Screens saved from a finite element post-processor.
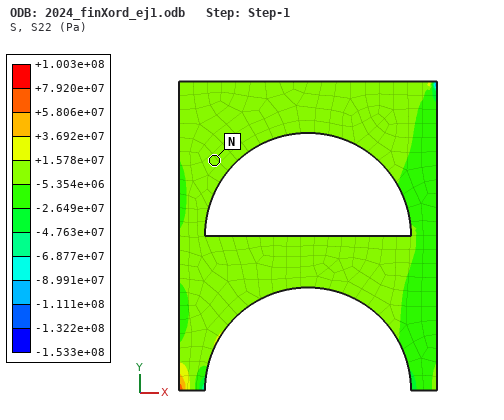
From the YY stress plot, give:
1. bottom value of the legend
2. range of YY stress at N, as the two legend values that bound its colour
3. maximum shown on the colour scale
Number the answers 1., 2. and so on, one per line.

1. -1.533e+08 Pa
2. -5.354e+06 to +1.578e+07 Pa
3. +1.003e+08 Pa
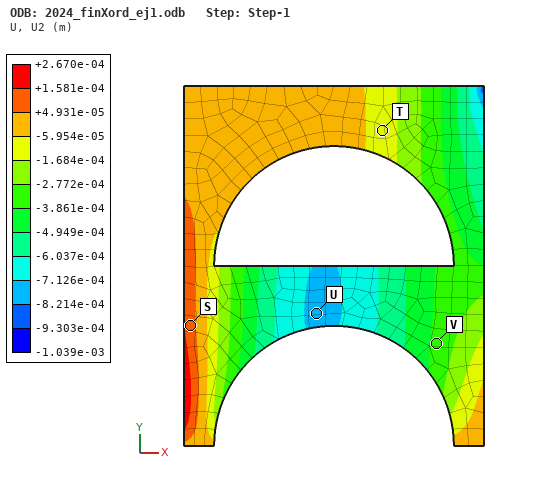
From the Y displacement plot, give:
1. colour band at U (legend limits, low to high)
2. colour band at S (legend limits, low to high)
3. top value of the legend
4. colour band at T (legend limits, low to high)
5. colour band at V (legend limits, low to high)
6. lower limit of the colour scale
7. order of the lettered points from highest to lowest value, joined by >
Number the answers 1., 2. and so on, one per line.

1. -8.214e-04 to -7.126e-04 m
2. +4.931e-05 to +1.581e-04 m
3. +2.670e-04 m
4. -1.684e-04 to -5.954e-05 m
5. -3.861e-04 to -2.772e-04 m
6. -1.039e-03 m
7. S > T > V > U
